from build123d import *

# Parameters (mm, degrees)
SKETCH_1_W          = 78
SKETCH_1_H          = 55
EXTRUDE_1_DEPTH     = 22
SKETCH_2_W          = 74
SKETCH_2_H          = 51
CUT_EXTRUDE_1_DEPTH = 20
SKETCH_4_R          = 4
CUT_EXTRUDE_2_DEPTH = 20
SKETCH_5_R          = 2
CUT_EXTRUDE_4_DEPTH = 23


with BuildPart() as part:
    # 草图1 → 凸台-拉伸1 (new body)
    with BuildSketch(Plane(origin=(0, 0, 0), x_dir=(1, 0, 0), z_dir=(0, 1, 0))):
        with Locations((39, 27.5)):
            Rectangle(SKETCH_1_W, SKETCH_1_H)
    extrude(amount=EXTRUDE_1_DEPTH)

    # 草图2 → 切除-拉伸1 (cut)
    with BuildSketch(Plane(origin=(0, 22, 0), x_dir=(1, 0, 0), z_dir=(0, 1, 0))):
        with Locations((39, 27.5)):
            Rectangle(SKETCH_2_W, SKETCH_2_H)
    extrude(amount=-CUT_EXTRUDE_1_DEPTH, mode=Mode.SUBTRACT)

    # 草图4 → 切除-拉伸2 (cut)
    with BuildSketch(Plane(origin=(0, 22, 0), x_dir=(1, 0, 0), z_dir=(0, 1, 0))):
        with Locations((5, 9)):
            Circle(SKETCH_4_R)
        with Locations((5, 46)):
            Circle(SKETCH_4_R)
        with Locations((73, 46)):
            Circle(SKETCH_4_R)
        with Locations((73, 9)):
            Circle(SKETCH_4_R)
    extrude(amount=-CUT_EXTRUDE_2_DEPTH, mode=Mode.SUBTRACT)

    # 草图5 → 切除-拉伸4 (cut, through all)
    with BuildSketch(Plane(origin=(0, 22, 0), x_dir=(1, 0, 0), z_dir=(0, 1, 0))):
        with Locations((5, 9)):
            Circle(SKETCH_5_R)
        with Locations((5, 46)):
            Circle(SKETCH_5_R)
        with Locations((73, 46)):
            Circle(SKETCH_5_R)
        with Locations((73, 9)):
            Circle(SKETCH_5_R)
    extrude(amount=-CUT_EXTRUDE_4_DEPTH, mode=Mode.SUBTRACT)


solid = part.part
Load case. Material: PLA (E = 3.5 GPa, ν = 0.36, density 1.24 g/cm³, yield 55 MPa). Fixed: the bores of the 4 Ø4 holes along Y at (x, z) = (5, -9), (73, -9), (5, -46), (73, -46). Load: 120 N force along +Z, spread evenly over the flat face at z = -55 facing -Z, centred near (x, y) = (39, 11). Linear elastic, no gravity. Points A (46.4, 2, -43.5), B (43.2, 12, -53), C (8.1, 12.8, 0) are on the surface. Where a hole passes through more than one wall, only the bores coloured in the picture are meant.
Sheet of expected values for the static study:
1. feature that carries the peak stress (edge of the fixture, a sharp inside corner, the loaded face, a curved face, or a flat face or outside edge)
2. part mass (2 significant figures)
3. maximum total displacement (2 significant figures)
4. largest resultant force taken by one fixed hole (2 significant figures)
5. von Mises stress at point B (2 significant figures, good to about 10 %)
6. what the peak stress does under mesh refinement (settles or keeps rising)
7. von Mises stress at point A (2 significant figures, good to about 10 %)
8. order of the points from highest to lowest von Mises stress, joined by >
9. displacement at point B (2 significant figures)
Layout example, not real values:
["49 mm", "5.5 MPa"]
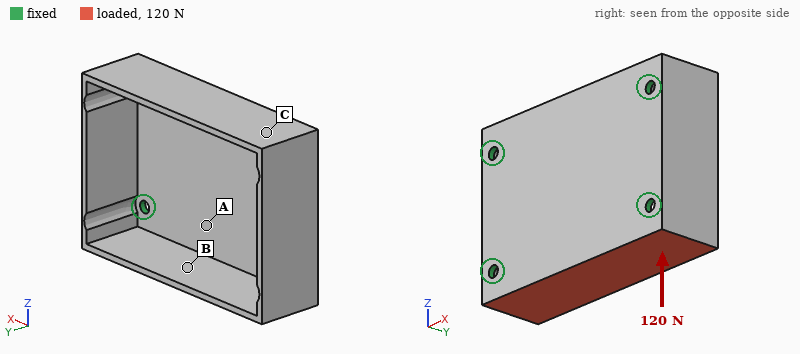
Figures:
["a sharp inside corner", "23 g", "1.0 mm", "40 N", "3.6 MPa", "keeps rising", "6.7 MPa", "A > B > C", "0.49 mm"]
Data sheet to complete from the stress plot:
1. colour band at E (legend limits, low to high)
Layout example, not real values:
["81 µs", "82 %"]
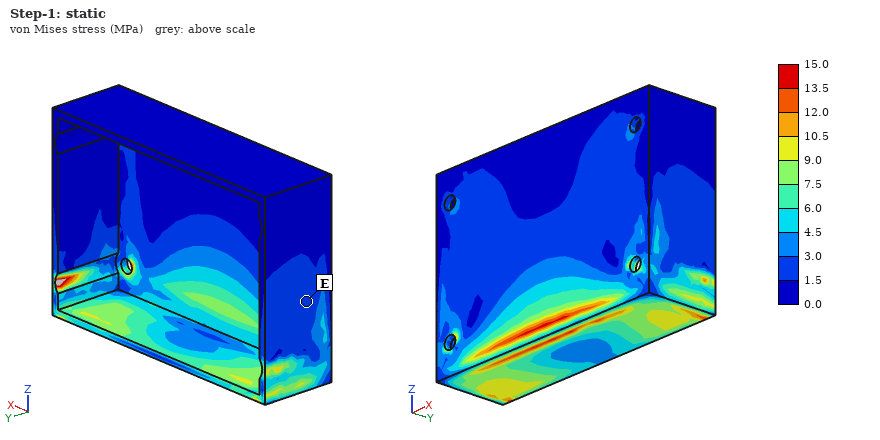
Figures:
["1.5 to 3.0 MPa"]
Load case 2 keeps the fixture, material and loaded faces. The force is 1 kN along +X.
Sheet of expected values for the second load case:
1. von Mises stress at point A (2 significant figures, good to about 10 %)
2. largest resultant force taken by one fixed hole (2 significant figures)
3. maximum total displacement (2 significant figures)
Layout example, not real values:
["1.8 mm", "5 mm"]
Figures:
["7.0 MPa", "480 N", "0.23 mm"]
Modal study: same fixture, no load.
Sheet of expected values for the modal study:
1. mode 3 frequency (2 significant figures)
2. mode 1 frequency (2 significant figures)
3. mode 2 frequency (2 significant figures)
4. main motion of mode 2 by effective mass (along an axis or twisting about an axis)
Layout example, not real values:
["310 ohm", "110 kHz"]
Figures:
["1400 Hz", "970 Hz", "1200 Hz", "along Z"]
